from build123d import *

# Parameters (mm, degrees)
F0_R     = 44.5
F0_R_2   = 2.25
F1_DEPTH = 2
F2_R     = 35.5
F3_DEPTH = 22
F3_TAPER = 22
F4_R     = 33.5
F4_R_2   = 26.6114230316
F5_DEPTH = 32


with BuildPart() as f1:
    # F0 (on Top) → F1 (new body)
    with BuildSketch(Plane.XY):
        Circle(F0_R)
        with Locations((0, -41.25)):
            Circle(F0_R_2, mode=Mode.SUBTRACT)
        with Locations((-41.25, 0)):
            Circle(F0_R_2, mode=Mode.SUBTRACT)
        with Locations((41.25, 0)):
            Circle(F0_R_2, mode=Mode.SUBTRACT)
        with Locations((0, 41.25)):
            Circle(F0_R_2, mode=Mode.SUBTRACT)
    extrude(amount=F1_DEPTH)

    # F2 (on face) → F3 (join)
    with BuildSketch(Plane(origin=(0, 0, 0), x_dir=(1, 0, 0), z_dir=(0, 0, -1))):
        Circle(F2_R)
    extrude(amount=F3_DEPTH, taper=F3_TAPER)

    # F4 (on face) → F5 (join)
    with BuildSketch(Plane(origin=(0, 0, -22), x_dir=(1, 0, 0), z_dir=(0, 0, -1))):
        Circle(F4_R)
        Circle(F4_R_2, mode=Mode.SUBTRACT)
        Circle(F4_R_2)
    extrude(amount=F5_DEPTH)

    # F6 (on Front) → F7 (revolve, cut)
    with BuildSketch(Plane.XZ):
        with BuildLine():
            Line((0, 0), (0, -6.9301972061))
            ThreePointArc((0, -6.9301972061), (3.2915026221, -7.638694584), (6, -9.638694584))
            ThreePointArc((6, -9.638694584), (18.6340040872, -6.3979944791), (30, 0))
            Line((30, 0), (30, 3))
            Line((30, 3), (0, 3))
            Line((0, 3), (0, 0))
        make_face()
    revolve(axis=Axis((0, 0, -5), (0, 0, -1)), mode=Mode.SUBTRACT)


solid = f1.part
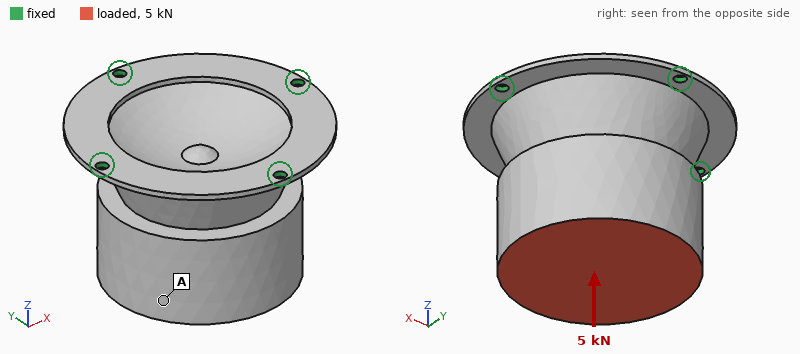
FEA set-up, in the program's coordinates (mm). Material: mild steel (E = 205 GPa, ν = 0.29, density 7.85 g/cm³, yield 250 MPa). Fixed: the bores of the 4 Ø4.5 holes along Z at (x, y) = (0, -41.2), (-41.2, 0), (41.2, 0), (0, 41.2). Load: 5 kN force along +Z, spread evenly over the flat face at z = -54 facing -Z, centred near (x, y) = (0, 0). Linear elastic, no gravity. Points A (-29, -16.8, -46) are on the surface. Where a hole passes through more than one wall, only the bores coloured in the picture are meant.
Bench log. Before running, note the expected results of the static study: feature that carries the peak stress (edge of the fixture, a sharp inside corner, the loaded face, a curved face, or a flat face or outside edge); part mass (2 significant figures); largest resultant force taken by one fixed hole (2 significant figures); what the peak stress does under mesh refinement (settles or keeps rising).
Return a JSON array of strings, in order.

["edge of the fixture", "1.4 kg", "1.6 kN", "keeps rising"]
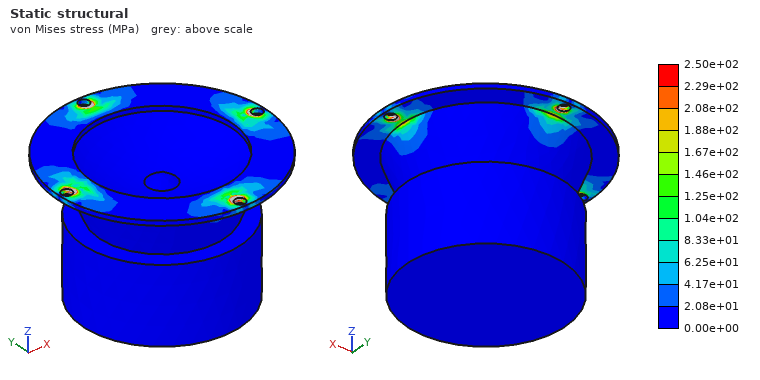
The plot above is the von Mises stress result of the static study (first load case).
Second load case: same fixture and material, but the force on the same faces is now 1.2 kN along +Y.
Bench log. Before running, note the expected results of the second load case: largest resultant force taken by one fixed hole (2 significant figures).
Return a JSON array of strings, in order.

["1.1 kN"]
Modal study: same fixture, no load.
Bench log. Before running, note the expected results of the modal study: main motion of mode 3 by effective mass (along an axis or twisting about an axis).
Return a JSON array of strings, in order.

["along Z"]
